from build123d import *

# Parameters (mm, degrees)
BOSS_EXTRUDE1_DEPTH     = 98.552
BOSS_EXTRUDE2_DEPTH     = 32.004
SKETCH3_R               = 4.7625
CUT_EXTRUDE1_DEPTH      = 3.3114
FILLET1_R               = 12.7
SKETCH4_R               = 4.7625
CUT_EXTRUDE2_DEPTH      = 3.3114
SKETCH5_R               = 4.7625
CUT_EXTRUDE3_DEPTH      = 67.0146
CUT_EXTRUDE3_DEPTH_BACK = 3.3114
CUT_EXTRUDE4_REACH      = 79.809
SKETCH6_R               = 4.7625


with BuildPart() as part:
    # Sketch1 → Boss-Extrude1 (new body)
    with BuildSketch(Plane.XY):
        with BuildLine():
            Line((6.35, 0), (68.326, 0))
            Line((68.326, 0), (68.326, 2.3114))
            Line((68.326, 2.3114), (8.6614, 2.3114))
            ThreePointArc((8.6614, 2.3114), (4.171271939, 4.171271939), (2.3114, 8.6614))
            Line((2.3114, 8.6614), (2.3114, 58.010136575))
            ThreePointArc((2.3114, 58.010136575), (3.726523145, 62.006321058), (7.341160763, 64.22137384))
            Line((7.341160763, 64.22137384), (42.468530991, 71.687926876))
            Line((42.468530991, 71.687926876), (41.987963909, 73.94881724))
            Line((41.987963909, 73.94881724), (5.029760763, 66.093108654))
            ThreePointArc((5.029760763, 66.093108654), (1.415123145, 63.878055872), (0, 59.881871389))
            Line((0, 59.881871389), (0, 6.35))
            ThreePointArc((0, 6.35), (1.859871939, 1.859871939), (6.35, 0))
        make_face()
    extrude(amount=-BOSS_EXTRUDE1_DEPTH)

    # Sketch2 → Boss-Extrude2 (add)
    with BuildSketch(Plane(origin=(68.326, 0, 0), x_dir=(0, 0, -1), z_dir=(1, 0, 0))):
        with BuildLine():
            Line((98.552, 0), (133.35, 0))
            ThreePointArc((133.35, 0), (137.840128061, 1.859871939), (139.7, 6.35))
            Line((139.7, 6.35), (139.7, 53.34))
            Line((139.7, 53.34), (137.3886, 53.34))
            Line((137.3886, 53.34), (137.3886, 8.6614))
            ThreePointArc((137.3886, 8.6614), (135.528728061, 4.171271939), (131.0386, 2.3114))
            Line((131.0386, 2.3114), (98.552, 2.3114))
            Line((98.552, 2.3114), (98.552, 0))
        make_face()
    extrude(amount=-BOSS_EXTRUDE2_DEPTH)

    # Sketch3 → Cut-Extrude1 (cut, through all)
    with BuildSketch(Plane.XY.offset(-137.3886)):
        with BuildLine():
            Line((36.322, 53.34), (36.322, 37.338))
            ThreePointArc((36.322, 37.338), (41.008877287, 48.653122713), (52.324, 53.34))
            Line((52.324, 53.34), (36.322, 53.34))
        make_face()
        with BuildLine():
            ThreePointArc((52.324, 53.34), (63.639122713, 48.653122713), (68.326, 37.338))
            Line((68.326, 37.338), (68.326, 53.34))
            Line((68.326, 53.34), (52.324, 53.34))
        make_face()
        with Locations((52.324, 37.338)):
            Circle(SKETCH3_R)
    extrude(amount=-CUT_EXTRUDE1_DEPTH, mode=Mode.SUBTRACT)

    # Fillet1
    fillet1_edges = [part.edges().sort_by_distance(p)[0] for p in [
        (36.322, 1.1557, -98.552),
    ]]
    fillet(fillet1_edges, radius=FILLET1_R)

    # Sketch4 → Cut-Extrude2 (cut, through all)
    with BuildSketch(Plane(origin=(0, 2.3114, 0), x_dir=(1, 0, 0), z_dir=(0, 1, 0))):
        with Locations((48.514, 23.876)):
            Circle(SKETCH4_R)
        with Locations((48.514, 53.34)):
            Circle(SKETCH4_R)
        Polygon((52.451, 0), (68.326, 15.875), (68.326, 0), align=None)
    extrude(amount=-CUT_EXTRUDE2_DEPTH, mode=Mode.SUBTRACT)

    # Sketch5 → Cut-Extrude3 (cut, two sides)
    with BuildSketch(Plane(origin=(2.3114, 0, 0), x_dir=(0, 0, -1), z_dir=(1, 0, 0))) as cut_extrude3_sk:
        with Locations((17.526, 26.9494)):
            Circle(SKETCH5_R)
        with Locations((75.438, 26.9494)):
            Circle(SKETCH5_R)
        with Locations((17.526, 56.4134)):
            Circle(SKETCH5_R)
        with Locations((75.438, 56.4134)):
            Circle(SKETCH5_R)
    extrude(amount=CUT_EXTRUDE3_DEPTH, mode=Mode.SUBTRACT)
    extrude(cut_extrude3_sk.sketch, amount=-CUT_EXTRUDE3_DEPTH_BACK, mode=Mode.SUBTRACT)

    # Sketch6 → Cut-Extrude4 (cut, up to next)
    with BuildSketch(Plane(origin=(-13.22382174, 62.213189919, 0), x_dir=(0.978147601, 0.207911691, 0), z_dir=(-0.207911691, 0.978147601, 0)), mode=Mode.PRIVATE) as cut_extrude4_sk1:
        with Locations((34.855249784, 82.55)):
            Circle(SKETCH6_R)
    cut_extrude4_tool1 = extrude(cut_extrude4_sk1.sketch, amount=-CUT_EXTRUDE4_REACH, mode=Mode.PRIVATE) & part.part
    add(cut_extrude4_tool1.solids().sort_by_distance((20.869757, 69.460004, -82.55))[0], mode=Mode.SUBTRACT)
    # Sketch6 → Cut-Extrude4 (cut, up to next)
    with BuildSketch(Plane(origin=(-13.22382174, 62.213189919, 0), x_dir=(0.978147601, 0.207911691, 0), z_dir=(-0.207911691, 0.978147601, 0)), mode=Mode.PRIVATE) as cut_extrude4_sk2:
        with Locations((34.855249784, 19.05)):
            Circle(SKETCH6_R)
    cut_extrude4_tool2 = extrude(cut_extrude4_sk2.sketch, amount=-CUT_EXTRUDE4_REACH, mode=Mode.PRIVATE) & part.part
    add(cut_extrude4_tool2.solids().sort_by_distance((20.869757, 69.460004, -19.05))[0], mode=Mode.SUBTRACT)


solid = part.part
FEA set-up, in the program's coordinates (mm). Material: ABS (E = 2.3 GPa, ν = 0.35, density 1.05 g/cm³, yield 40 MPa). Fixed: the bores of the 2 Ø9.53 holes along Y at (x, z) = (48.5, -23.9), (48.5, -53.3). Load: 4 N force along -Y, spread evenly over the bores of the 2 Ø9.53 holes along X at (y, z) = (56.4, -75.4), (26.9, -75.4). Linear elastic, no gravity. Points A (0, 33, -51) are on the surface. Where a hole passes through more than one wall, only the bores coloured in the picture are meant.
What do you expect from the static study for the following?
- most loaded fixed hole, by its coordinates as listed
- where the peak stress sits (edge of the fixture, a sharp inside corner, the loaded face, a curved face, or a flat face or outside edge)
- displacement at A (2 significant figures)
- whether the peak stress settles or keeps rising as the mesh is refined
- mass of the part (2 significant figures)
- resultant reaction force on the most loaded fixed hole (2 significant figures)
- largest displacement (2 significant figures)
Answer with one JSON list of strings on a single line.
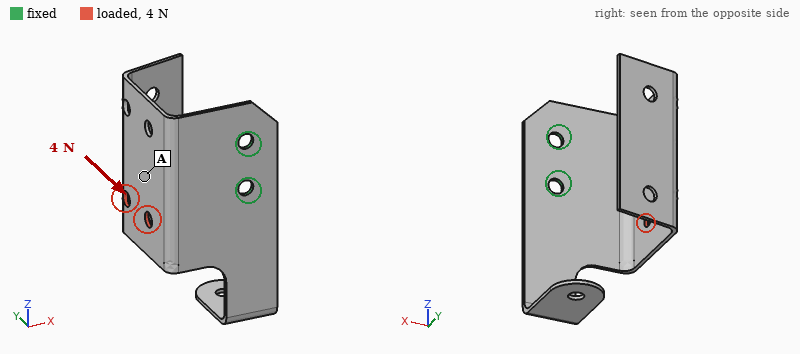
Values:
["(48.5, -53.3)", "edge of the fixture", "0.92 mm", "keeps rising", "46 g", "4.9 N", "1.8 mm"]
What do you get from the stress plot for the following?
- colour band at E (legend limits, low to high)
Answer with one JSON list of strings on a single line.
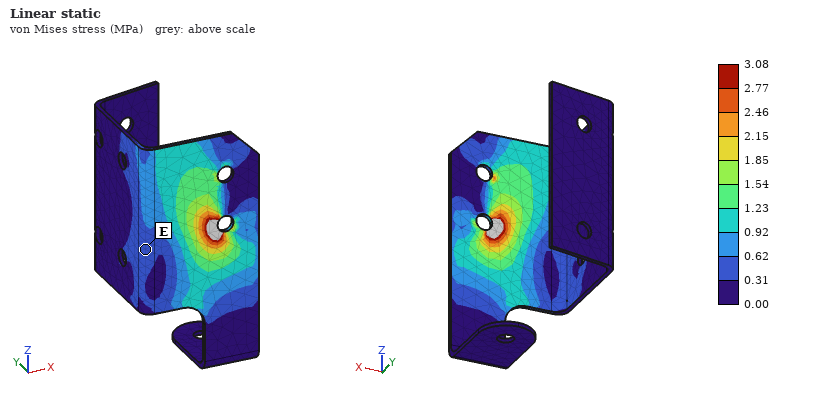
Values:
["0.31 to 0.62 MPa"]
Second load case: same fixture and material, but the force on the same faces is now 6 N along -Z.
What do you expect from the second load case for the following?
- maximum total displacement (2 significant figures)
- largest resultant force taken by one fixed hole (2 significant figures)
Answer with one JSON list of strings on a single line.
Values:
["1.7 mm", "9.5 N"]
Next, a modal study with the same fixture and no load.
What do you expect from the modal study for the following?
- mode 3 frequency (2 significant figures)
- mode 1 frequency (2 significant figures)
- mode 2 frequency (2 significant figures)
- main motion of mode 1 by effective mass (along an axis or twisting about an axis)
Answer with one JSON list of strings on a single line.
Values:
["65 Hz", "39 Hz", "51 Hz", "along X"]
